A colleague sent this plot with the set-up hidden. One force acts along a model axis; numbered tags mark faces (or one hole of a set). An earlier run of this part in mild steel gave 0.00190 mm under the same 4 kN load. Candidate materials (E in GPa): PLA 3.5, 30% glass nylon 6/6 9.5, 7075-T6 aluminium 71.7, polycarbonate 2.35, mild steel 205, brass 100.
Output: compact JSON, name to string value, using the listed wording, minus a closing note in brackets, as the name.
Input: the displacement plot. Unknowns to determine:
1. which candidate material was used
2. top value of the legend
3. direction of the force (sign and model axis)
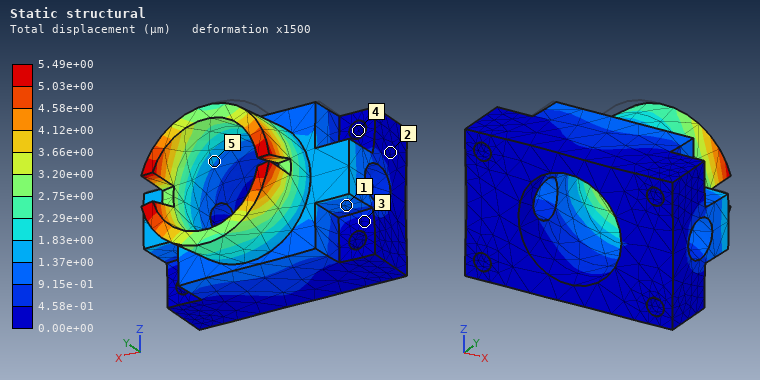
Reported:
{"which candidate material was used": "7075-T6 aluminium", "top value of the legend": "5.49e+00 µm", "direction of the force": "+X"}
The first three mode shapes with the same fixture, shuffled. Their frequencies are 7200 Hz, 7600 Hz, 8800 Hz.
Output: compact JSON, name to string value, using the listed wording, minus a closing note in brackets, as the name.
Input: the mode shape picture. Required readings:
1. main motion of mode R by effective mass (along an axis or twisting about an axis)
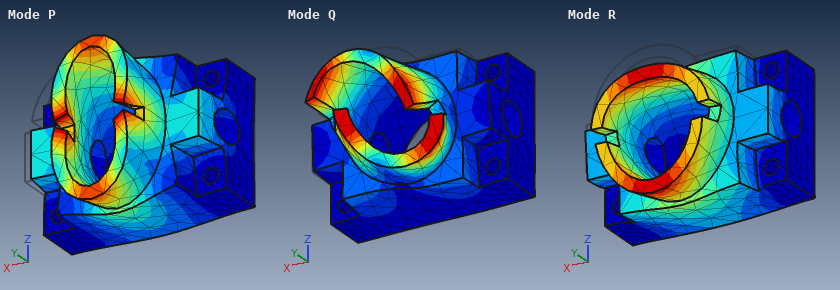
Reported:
{"main motion of mode R by effective mass": "along Z"}
